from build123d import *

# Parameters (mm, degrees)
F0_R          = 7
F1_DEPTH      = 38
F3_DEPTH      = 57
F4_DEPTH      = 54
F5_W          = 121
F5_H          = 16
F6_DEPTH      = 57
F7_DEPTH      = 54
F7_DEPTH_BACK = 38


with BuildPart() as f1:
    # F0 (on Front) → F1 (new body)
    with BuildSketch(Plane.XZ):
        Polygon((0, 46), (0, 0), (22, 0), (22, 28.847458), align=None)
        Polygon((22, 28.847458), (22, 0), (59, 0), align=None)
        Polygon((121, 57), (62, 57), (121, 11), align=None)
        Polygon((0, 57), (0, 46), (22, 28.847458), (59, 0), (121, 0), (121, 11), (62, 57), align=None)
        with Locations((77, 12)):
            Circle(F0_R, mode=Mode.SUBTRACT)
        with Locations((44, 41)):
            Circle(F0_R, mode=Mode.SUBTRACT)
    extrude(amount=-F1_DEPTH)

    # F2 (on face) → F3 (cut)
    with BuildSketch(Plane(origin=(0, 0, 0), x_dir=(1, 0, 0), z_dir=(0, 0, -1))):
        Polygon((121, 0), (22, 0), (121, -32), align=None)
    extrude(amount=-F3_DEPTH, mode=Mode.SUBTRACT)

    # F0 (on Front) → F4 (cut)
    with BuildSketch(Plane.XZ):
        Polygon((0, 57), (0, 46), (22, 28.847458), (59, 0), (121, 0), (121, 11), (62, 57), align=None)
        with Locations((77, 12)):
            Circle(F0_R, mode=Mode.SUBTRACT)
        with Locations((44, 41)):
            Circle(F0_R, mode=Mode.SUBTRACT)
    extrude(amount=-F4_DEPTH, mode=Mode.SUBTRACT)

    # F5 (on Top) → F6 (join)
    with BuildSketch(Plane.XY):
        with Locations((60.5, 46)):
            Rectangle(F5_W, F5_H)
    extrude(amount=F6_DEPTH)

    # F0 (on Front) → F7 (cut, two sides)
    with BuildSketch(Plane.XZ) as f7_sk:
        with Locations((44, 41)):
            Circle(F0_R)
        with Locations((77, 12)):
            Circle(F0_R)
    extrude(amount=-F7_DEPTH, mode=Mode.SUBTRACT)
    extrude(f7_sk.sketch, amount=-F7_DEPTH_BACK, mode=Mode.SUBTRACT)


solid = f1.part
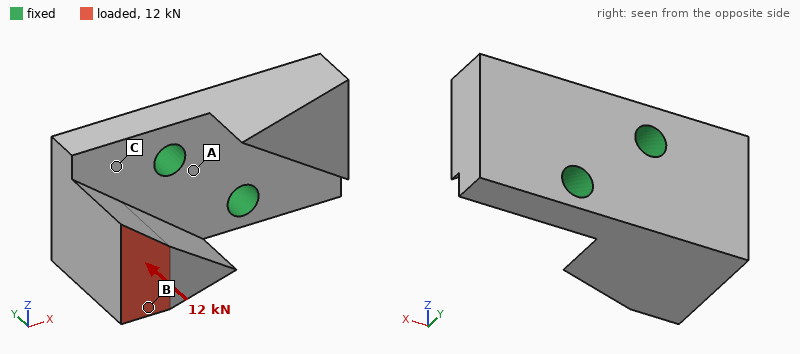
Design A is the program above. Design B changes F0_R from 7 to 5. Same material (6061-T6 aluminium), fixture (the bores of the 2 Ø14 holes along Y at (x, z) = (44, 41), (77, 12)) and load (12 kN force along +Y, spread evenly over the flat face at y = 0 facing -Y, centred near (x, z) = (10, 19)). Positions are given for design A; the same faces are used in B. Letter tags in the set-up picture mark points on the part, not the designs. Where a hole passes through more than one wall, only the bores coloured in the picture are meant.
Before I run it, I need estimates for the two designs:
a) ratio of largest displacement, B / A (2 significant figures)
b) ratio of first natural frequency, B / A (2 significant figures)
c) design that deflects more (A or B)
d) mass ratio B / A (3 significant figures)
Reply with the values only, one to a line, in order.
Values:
1.2
0.92
B
1.01
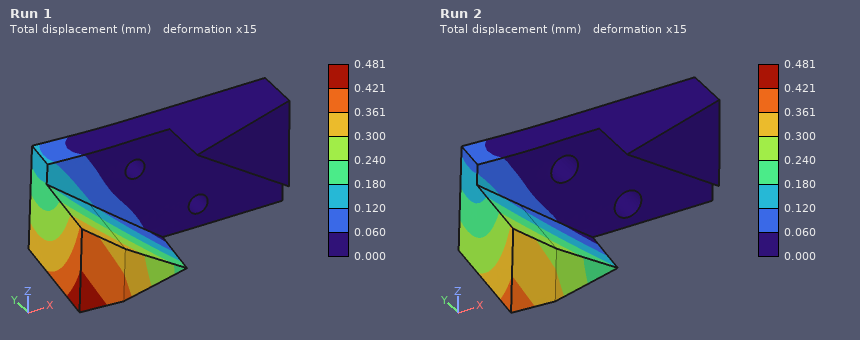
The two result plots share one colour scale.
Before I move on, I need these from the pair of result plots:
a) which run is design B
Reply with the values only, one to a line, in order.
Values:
Run 1
